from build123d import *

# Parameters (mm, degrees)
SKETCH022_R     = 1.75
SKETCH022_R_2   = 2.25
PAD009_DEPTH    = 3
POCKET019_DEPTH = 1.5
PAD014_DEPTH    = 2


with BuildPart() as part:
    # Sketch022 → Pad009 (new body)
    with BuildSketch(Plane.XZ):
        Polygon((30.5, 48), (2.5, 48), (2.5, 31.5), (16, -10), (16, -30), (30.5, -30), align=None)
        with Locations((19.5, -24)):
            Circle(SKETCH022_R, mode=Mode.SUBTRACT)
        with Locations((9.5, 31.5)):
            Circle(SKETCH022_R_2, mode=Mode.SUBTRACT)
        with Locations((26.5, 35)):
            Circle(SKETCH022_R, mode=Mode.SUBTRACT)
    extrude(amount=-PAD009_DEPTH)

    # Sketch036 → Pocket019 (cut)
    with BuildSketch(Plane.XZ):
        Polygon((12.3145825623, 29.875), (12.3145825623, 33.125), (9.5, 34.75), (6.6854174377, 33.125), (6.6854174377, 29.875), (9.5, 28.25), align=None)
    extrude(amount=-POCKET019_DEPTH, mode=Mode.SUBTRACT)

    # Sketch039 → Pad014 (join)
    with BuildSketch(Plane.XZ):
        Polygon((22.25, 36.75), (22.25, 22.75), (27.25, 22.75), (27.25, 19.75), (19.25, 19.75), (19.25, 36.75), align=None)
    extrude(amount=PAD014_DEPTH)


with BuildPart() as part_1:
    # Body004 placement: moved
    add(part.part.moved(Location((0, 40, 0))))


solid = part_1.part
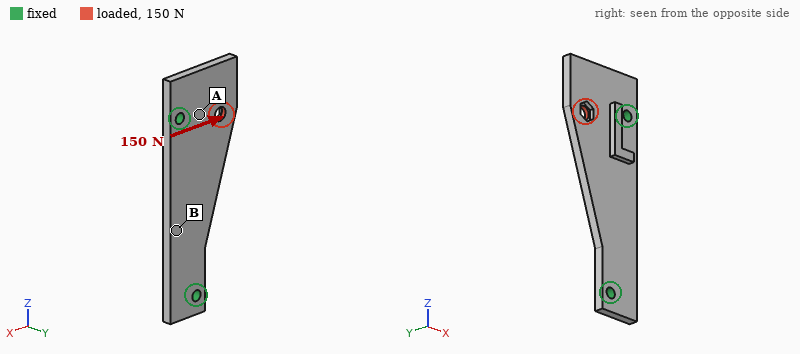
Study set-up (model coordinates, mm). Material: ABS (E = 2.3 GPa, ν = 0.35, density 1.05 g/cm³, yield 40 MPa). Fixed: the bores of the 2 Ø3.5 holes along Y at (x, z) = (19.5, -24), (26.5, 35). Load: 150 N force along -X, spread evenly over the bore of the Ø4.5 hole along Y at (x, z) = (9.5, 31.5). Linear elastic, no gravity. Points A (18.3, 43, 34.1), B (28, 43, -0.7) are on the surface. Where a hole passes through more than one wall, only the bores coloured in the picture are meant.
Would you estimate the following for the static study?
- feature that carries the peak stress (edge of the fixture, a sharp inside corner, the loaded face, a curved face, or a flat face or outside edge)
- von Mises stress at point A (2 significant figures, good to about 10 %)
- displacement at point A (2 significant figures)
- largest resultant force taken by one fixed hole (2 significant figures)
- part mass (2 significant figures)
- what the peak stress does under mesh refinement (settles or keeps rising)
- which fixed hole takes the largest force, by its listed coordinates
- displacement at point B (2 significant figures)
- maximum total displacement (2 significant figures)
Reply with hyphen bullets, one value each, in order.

- edge of the fixture
- 6.3 MPa
- 0.039 mm
- 140 N
- 5.2 g
- keeps rising
- (26.5, 35)
- 0.038 mm
- 0.22 mm
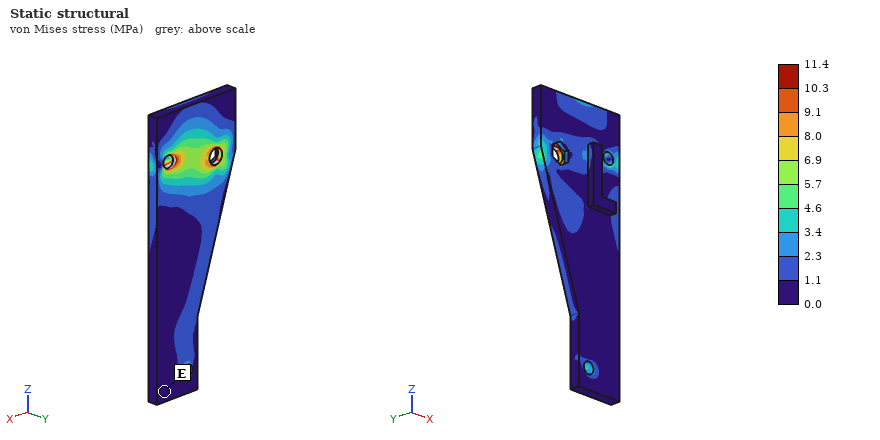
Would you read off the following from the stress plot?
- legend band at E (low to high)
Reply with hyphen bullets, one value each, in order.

- 0.0 to 1.1 MPa
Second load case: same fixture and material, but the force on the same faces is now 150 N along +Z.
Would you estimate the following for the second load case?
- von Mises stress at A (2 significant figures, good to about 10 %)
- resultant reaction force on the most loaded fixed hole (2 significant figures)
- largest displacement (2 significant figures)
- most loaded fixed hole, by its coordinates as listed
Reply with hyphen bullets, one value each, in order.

- 3.2 MPa
- 96 N
- 0.19 mm
- (26.5, 35)
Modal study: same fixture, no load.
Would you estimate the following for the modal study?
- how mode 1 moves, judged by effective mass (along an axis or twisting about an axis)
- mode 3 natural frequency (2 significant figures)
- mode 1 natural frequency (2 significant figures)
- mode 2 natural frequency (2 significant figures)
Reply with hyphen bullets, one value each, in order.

- along Y
- 2200 Hz
- 1100 Hz
- 1300 Hz
